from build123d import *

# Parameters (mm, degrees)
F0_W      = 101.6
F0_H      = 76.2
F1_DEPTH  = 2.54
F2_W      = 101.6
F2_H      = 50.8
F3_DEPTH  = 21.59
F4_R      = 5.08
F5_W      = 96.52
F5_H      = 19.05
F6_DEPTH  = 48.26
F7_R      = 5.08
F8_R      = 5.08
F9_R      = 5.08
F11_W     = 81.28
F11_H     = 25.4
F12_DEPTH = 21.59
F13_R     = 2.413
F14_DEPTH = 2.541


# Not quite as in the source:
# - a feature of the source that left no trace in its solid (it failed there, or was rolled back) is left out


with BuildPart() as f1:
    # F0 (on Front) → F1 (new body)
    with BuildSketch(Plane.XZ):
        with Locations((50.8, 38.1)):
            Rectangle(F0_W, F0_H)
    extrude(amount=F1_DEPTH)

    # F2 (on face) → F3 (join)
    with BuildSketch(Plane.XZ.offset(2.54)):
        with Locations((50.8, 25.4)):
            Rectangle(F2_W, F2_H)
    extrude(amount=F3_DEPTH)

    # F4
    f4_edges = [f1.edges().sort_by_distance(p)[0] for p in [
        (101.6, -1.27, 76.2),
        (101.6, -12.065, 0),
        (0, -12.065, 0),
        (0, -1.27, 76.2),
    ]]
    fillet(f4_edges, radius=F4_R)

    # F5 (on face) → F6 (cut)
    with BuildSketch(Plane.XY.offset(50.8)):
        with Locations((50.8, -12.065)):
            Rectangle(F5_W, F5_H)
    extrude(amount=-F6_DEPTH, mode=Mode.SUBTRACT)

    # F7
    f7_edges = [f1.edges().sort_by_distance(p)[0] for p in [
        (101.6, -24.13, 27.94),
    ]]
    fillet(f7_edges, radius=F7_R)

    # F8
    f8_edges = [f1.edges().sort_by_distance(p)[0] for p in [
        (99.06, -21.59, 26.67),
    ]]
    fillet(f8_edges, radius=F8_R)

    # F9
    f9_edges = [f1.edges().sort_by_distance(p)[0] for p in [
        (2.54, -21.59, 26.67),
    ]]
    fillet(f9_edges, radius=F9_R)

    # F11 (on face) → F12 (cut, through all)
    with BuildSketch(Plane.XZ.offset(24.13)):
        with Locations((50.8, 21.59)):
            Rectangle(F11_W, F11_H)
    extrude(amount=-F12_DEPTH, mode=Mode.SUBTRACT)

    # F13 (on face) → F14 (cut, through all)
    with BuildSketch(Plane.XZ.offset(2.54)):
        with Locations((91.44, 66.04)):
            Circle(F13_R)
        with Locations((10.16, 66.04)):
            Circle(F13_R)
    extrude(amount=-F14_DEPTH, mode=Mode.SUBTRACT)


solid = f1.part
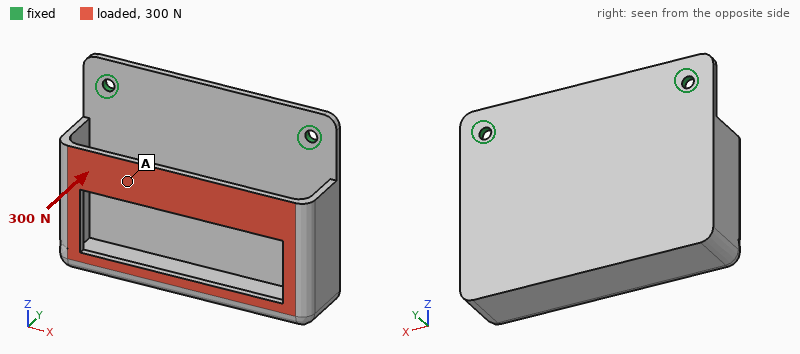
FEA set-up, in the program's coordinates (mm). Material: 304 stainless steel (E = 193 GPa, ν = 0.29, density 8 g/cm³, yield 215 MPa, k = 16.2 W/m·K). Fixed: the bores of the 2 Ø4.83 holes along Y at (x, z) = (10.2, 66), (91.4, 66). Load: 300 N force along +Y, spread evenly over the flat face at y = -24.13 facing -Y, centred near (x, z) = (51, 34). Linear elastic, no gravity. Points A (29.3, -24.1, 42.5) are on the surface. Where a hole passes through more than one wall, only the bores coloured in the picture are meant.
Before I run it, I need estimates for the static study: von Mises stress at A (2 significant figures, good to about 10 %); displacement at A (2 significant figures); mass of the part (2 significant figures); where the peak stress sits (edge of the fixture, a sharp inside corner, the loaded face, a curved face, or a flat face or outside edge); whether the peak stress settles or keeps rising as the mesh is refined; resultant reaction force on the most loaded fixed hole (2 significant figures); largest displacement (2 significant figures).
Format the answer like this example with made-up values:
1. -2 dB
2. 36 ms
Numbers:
1. 22 MPa
2. 0.26 mm
3. 290 g
4. edge of the fixture
5. keeps rising
6. 150 N
7. 0.45 mm
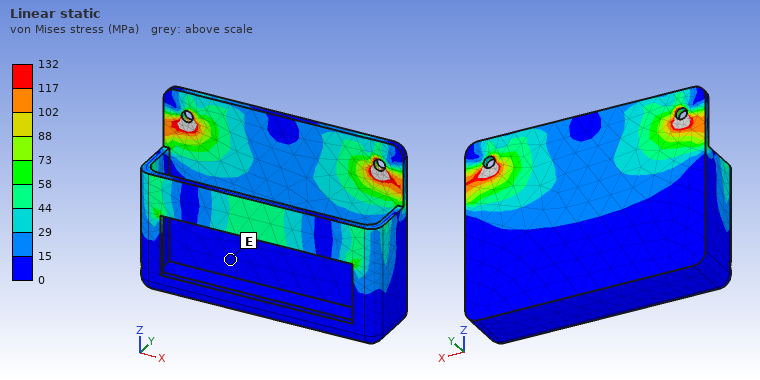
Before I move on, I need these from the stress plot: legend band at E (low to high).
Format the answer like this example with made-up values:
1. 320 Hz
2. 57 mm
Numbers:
1. 0 to 15 MPa
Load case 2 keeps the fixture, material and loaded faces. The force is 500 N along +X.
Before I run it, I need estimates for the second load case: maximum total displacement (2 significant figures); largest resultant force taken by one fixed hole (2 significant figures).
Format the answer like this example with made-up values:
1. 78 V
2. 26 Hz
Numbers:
1. 0.19 mm
2. 330 N
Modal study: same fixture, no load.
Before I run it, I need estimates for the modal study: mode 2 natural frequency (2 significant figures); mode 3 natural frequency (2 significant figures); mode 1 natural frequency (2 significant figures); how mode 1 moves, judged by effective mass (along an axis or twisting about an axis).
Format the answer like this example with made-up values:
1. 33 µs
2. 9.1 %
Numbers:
1. 710 Hz
2. 1300 Hz
3. 240 Hz
4. along Y
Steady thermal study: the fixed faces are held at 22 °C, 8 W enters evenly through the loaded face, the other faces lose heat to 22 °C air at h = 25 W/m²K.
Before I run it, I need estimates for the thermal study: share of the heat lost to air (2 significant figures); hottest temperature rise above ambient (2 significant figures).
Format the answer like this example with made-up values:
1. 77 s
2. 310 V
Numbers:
1. 93 %
2. 71 K
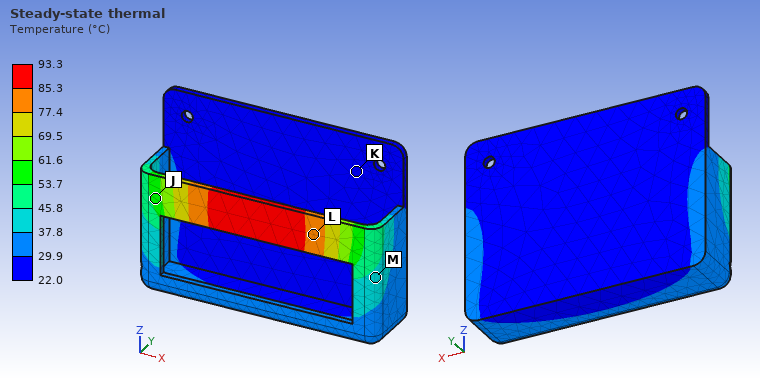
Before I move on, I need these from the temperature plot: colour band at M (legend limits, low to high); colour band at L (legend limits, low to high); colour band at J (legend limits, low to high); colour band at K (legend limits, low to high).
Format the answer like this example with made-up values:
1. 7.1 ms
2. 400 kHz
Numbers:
1. 37.8 to 45.8 °C
2. 77.4 to 85.3 °C
3. 53.7 to 61.6 °C
4. 22.0 to 29.9 °C
